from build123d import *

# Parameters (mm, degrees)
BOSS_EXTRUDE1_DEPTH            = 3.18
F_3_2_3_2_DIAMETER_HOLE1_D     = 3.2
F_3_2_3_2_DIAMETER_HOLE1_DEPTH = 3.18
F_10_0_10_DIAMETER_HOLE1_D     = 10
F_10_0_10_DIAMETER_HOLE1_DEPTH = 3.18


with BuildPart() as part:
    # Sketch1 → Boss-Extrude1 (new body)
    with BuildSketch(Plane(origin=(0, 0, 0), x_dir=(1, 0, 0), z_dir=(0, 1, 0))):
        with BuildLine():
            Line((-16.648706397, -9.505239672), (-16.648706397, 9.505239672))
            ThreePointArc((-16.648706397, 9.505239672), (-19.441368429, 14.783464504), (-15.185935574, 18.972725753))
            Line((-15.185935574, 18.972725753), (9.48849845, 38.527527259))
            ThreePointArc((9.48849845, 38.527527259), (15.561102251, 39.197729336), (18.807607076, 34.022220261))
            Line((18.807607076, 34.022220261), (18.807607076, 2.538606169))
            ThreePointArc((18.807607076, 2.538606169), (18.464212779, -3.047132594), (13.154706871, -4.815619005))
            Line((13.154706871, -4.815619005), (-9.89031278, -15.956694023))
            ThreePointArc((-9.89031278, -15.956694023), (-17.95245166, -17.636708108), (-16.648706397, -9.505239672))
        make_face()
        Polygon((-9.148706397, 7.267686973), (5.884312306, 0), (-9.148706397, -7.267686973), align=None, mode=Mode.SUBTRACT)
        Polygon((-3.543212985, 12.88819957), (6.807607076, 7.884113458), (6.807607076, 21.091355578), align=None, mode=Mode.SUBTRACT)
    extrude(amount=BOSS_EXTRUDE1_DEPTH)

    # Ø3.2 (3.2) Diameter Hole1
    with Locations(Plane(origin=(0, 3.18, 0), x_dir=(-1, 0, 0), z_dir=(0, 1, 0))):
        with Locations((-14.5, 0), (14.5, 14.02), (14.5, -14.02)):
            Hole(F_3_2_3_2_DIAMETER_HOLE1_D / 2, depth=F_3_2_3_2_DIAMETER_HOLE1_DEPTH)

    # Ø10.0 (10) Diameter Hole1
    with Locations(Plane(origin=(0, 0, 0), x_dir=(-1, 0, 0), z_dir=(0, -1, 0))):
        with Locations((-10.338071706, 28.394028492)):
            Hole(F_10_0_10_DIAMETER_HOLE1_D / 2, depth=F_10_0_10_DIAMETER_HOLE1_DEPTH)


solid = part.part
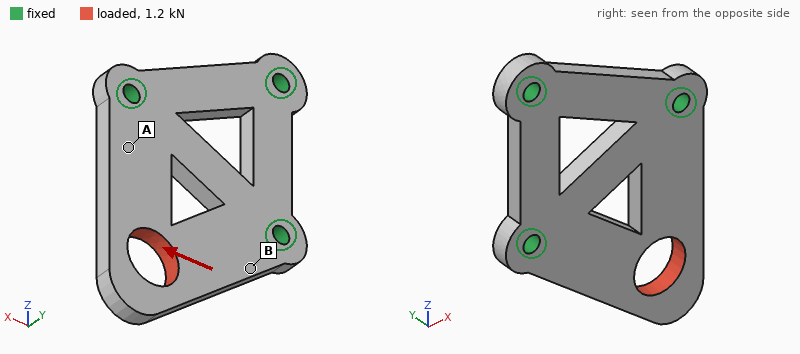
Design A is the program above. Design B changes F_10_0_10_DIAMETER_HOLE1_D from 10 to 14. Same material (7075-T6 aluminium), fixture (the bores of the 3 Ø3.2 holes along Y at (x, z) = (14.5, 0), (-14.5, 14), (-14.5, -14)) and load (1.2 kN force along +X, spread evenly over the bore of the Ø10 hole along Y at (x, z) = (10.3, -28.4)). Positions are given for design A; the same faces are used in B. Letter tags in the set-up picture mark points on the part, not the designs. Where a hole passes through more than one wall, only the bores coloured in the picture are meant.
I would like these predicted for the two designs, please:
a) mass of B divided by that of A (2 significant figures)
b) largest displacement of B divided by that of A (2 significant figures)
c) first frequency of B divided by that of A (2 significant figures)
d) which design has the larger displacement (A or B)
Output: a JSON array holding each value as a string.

["0.94", "2.9", "1.1", "B"]
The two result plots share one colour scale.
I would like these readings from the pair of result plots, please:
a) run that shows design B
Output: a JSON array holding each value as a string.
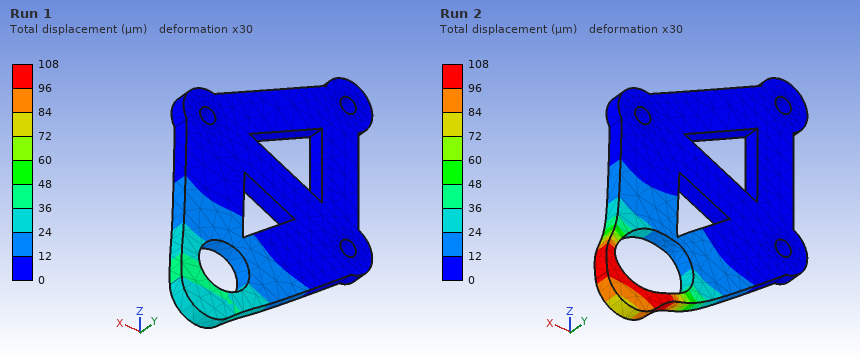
["Run 2"]
